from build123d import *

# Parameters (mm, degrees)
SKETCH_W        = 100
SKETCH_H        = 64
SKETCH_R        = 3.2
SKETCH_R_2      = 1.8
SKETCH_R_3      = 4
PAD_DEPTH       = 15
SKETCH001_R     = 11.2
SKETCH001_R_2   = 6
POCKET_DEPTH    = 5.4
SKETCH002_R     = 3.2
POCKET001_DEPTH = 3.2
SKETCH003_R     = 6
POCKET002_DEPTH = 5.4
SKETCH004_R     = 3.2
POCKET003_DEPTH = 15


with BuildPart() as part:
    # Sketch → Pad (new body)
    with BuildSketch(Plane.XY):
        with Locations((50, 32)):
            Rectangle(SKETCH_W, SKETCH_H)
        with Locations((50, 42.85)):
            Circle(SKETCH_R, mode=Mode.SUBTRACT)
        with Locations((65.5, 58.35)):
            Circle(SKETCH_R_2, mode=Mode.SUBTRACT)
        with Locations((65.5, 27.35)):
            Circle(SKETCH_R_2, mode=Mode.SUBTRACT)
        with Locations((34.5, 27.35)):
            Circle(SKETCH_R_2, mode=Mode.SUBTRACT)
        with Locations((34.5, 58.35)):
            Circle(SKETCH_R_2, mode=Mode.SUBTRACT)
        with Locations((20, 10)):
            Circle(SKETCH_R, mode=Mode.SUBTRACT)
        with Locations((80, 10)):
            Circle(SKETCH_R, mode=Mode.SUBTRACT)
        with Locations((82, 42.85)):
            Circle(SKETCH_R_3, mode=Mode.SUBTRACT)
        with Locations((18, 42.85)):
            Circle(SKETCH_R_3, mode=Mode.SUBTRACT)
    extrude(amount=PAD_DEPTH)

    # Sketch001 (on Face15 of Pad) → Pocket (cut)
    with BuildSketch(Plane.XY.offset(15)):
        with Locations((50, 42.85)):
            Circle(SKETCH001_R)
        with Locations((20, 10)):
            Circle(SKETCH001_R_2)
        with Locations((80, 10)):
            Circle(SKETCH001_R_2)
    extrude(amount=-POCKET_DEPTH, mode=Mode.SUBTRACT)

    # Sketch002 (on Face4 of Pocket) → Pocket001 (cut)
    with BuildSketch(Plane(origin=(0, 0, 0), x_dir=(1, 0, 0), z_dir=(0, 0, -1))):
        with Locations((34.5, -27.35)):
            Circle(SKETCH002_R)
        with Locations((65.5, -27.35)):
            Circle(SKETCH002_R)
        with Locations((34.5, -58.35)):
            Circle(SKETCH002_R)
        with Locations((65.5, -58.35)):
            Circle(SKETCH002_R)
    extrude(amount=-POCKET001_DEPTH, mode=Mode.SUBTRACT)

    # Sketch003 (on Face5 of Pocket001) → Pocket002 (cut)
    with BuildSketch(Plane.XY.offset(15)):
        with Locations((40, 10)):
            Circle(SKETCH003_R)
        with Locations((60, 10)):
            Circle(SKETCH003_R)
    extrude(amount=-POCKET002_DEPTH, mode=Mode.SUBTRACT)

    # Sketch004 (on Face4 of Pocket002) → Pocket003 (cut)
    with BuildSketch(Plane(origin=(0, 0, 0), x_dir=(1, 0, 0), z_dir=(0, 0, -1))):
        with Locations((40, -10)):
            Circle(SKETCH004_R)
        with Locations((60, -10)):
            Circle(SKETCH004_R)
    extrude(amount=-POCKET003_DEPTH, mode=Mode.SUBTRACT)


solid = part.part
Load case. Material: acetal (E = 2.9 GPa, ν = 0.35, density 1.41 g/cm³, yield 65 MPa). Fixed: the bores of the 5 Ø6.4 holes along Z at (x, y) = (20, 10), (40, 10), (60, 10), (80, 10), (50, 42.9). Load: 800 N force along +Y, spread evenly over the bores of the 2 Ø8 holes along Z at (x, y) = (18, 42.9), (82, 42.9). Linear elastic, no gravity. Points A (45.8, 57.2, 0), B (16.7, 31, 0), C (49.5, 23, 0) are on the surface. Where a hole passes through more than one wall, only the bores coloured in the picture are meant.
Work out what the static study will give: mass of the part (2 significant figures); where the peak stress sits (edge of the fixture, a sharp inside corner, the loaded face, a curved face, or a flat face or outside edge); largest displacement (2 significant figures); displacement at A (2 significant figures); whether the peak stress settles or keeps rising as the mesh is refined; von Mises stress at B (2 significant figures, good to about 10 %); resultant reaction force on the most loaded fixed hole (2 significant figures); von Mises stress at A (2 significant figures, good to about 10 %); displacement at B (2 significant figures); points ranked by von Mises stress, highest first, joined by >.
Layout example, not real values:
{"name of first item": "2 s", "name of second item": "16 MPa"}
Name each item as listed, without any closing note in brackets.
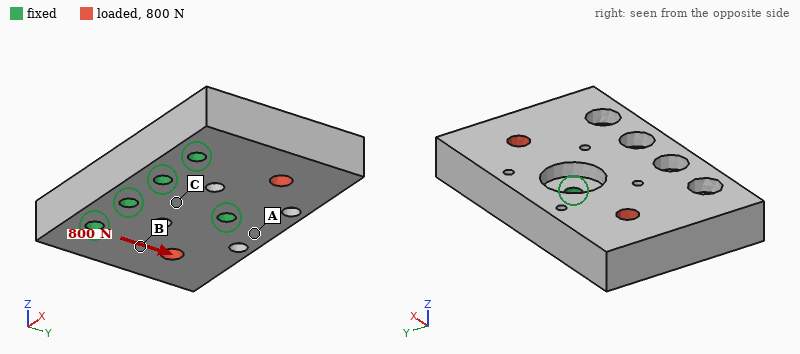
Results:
{"mass of the part": "120 g", "where the peak stress sits": "edge of the fixture", "largest displacement": "16 µm", "displacement at A": "3.4 µm", "whether the peak stress settles or keeps rising as the mesh is refined": "keeps rising", "von Mises stress at B": "1.1 MPa", "resultant reaction force on the most loaded fixed hole": "240 N", "von Mises stress at A": "0.65 MPa", "displacement at B": "8.1 µm", "points ranked by von Mises stress, highest first, joined by >": "B > A > C"}
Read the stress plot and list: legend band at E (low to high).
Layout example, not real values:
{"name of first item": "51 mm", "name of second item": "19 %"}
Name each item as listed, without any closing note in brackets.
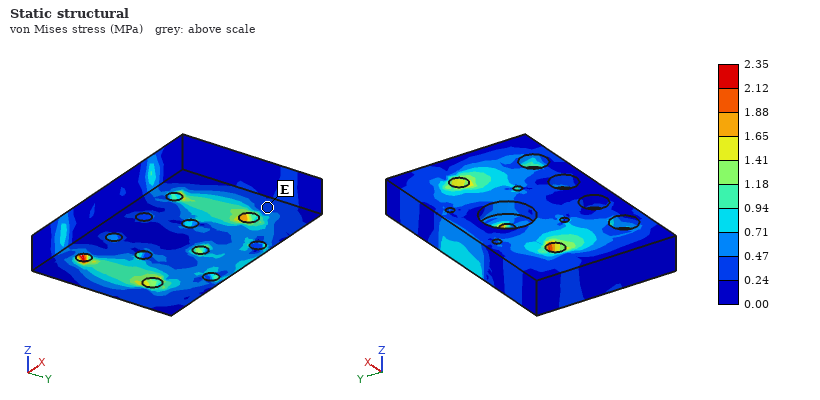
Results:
{"legend band at E": "0.24 to 0.47 MPa"}
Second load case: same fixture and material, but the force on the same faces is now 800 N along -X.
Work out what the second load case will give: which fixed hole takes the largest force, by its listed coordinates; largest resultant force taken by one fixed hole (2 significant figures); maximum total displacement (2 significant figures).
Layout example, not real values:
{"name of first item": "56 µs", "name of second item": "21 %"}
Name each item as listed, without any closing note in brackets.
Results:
{"which fixed hole takes the largest force, by its listed coordinates": "(50, 42.9)", "largest resultant force taken by one fixed hole": "540 N", "maximum total displacement": "23 µm"}
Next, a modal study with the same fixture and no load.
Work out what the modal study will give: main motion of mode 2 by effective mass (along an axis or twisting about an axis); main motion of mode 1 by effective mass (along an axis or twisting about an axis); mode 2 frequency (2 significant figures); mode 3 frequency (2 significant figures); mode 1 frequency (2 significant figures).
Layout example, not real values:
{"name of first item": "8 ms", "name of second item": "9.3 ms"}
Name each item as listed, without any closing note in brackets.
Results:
{"main motion of mode 2 by effective mass": "along Z", "main motion of mode 1 by effective mass": "twisting about Y", "mode 2 frequency": "1600 Hz", "mode 3 frequency": "3700 Hz", "mode 1 frequency": "1400 Hz"}
